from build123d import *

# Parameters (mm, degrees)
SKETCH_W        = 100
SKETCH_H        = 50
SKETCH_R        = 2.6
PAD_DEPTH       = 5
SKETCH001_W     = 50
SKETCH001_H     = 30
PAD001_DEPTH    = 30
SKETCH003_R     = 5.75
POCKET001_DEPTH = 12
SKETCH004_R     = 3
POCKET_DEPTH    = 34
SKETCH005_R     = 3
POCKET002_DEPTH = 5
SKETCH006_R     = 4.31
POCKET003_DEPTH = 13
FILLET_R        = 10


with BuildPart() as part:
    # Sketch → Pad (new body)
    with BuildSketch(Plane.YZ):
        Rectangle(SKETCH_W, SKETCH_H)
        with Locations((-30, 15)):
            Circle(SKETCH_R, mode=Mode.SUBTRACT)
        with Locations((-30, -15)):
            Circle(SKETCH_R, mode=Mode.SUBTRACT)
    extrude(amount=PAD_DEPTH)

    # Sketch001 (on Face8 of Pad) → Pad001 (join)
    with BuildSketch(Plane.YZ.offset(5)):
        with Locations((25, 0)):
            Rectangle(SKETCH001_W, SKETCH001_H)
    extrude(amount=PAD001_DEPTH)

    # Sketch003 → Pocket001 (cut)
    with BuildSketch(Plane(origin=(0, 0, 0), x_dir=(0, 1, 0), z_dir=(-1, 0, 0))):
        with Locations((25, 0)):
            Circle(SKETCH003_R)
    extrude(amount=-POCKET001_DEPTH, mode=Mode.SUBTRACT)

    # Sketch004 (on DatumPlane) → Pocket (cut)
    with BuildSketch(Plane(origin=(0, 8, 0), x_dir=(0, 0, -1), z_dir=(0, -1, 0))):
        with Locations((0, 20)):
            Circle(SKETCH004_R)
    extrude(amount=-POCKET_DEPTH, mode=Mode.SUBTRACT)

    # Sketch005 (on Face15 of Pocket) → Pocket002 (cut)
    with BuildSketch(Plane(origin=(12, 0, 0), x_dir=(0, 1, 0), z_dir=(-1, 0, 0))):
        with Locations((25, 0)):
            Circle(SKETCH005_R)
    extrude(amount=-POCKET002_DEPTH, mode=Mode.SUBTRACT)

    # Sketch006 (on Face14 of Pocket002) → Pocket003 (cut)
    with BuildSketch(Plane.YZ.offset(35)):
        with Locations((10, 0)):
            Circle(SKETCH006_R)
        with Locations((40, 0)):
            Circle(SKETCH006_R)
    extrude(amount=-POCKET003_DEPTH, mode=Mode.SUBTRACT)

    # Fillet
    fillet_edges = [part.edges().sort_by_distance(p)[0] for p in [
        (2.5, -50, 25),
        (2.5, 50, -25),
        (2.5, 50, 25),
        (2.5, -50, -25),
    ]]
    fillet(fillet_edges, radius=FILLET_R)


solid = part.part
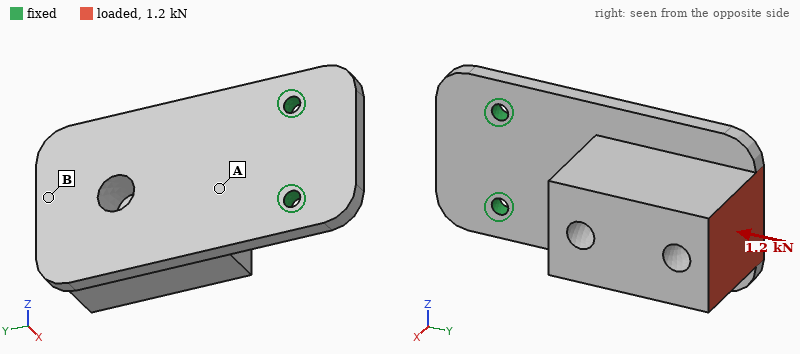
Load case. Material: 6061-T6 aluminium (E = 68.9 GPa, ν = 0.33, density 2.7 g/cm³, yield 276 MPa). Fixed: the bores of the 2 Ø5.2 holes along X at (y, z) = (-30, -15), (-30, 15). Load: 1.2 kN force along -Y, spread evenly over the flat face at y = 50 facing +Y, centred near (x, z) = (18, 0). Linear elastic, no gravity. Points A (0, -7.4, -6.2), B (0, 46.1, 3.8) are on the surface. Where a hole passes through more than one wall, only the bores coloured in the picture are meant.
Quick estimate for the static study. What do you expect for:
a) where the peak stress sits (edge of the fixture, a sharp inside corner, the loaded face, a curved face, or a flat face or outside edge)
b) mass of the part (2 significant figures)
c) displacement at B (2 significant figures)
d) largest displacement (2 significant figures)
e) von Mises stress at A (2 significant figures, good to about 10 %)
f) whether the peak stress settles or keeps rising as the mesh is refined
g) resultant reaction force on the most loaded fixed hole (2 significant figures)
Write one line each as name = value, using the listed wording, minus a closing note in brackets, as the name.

where the peak stress sits = edge of the fixture
mass of the part = 180 g
displacement at B = 0.94 mm
largest displacement = 1.1 mm
von Mises stress at A = 73 MPa
whether the peak stress settles or keeps rising as the mesh is refined = keeps rising
resultant reaction force on the most loaded fixed hole = 610 N
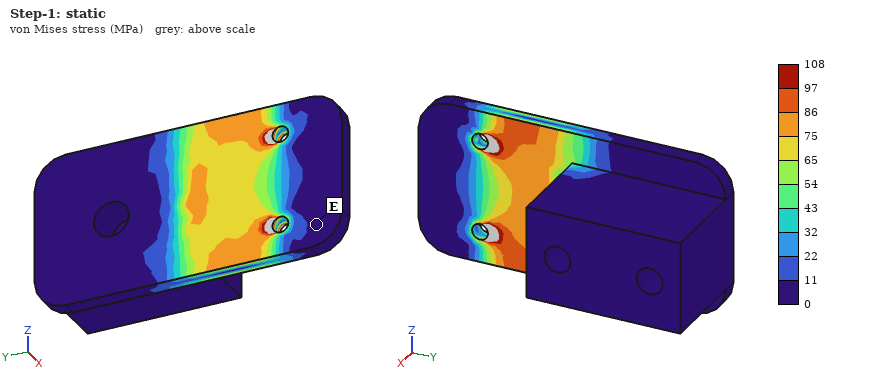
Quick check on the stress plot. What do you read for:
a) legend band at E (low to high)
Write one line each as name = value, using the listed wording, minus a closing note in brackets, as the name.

legend band at E = 0 to 11 MPa
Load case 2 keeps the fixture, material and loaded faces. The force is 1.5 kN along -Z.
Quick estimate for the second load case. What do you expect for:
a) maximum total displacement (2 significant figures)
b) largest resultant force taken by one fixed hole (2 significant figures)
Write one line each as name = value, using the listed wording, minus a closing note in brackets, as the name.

maximum total displacement = 0.31 mm
largest resultant force taken by one fixed hole = 3.8 kN
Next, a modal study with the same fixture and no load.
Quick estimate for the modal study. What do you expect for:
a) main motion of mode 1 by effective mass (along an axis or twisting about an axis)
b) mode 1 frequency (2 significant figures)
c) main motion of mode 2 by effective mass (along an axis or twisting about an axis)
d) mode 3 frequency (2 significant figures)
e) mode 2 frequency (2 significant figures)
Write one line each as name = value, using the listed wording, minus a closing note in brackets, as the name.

main motion of mode 1 by effective mass = along X
mode 1 frequency = 310 Hz
main motion of mode 2 by effective mass = along Z
mode 3 frequency = 2600 Hz
mode 2 frequency = 1200 Hz
